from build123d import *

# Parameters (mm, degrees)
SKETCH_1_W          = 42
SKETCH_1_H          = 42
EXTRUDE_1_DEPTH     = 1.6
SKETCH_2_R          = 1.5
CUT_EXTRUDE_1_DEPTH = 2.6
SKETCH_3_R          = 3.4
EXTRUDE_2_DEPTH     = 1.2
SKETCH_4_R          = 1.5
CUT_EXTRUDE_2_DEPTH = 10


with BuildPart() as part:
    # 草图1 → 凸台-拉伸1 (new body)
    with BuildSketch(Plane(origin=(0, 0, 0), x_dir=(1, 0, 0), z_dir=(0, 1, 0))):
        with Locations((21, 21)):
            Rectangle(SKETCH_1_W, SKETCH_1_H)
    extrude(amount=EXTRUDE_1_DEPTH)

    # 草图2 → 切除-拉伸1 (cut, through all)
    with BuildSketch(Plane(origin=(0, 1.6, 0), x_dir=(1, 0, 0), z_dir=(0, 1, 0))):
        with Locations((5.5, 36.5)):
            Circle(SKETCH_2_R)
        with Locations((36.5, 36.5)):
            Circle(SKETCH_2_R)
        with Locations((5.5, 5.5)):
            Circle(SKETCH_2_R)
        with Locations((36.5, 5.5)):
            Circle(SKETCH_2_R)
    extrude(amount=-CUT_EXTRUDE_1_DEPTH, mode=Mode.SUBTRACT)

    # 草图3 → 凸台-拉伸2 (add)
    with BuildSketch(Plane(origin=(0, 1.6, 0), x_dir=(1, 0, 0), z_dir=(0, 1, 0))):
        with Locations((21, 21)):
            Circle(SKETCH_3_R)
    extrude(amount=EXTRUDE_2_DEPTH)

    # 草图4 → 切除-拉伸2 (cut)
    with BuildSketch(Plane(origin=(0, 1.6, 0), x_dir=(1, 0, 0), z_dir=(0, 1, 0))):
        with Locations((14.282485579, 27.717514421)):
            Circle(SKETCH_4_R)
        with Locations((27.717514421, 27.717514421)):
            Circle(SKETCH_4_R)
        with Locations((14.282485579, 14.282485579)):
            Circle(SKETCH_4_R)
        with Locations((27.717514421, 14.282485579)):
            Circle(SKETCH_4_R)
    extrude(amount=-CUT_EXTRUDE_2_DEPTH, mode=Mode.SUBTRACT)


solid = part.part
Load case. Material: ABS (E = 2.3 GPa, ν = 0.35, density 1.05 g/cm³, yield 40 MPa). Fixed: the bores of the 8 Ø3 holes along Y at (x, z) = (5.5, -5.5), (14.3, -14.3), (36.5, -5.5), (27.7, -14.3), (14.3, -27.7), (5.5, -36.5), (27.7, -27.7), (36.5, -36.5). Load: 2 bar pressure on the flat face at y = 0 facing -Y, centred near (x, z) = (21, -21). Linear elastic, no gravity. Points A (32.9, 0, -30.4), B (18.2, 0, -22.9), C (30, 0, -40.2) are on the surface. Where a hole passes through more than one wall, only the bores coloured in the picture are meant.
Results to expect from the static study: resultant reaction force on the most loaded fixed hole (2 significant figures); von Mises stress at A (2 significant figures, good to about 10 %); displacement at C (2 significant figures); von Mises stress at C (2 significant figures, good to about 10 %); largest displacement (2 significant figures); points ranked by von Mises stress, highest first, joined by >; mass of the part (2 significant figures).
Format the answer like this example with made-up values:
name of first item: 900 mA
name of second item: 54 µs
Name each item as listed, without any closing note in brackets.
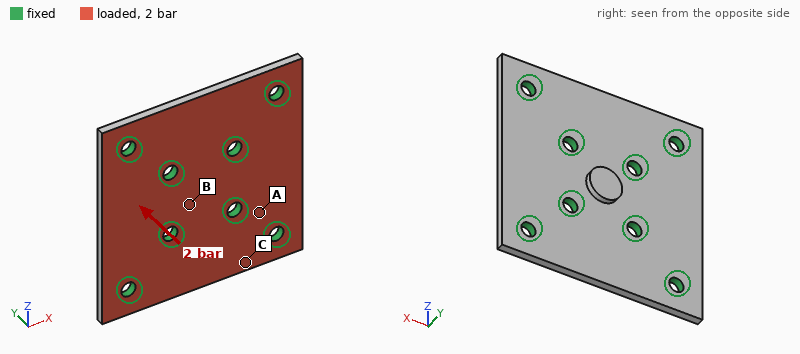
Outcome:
resultant reaction force on the most loaded fixed hole: 43 N
von Mises stress at A: 11 MPa
displacement at C: 0.15 mm
von Mises stress at C: 5.3 MPa
largest displacement: 0.37 mm
points ranked by von Mises stress, highest first, joined by >: A > C > B
mass of the part: 2.9 g
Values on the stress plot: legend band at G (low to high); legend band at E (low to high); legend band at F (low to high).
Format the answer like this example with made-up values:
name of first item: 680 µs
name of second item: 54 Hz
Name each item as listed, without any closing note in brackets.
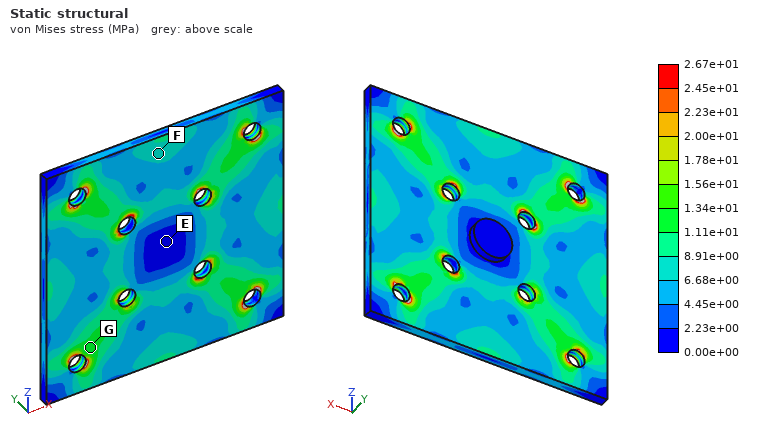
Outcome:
legend band at G: 1.11e+01 to 1.34e+01 MPa
legend band at E: 0.00e+00 to 2.23e+00 MPa
legend band at F: 6.68e+00 to 8.91e+00 MPa
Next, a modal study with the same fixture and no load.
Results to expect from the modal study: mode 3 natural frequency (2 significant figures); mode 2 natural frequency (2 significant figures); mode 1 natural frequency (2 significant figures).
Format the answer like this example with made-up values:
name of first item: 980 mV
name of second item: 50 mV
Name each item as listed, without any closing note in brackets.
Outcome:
mode 3 natural frequency: 3800 Hz
mode 2 natural frequency: 3800 Hz
mode 1 natural frequency: 3700 Hz
